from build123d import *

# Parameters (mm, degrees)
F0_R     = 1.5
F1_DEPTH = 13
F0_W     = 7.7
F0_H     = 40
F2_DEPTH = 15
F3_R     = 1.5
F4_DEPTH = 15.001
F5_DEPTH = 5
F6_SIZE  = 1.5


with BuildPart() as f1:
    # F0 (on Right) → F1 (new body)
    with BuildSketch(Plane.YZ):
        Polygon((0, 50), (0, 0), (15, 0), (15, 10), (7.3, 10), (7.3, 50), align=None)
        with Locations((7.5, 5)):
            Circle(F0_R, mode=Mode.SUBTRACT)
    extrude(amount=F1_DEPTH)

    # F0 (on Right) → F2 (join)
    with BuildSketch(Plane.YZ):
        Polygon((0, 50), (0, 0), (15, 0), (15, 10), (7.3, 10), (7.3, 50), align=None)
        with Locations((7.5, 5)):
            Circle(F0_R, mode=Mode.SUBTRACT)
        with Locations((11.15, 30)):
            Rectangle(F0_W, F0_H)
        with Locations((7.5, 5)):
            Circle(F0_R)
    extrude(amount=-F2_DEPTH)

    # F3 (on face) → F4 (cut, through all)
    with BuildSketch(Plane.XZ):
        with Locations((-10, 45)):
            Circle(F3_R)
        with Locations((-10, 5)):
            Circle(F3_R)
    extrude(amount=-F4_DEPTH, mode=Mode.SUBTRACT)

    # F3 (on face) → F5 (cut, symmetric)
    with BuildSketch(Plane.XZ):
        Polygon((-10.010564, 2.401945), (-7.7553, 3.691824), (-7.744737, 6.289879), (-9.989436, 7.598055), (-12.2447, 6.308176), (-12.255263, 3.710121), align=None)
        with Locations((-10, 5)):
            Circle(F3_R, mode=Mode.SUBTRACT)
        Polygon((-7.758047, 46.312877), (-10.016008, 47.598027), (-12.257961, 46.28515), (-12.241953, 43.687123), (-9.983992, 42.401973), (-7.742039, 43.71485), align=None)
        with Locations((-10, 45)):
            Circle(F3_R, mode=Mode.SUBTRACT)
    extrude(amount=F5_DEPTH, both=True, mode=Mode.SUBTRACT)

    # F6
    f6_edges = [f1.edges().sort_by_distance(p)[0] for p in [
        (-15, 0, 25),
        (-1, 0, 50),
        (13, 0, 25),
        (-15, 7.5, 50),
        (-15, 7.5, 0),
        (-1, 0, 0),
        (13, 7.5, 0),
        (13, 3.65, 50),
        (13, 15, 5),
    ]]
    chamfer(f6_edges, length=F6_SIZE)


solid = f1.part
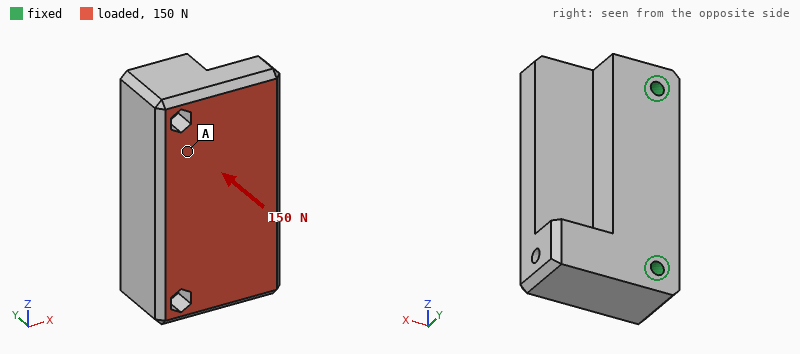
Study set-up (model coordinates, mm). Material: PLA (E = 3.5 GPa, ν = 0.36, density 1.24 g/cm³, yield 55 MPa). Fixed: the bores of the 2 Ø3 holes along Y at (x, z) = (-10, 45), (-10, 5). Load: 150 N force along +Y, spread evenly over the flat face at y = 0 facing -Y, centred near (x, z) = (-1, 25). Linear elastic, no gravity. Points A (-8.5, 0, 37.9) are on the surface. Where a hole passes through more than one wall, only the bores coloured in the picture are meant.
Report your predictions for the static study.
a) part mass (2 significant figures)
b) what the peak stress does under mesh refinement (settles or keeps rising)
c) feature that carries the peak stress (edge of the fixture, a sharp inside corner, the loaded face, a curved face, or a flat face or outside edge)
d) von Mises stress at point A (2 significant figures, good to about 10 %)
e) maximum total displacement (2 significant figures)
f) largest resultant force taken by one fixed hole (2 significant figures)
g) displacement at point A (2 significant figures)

20 g
keeps rising
edge of the fixture
0.71 MPa
37 µm
77 N
10 µm
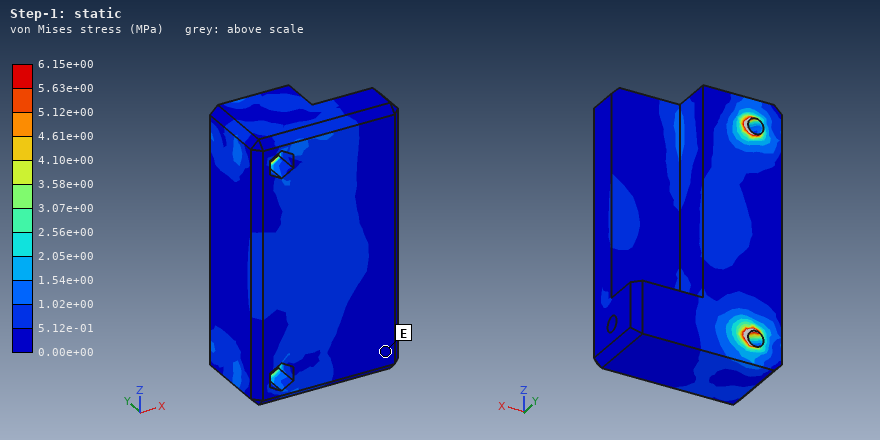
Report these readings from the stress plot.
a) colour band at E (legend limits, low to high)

0.00e+00 to 5.12e-01 MPa
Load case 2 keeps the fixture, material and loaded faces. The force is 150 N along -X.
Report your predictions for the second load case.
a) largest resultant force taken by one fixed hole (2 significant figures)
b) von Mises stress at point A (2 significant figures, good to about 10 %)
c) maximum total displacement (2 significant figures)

78 N
0.92 MPa
33 µm
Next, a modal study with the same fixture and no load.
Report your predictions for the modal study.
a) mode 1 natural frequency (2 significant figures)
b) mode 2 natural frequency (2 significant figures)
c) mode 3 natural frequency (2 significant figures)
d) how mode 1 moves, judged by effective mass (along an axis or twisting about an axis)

3300 Hz
5600 Hz
7300 Hz
along Y
